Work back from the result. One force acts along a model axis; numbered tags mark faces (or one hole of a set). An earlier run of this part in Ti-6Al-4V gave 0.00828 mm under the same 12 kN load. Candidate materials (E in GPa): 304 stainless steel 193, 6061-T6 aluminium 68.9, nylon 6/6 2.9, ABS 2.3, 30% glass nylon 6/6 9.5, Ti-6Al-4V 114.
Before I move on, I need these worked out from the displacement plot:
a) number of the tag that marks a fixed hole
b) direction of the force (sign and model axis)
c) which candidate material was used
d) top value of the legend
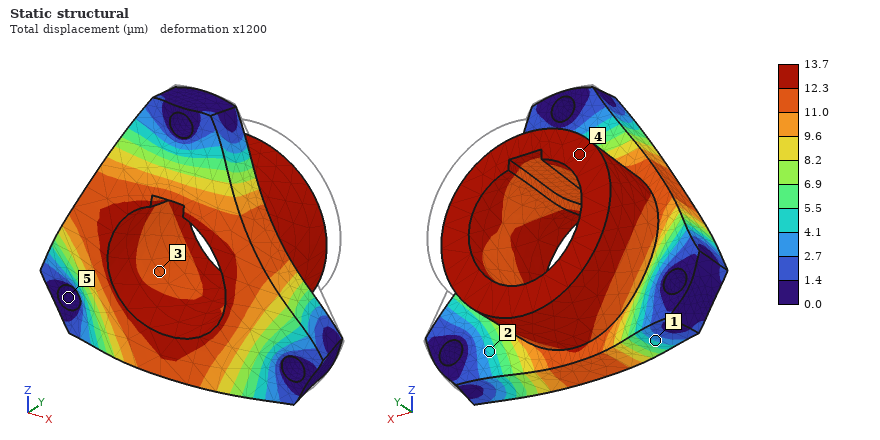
5
-Y
6061-T6 aluminium
13.7 µm
